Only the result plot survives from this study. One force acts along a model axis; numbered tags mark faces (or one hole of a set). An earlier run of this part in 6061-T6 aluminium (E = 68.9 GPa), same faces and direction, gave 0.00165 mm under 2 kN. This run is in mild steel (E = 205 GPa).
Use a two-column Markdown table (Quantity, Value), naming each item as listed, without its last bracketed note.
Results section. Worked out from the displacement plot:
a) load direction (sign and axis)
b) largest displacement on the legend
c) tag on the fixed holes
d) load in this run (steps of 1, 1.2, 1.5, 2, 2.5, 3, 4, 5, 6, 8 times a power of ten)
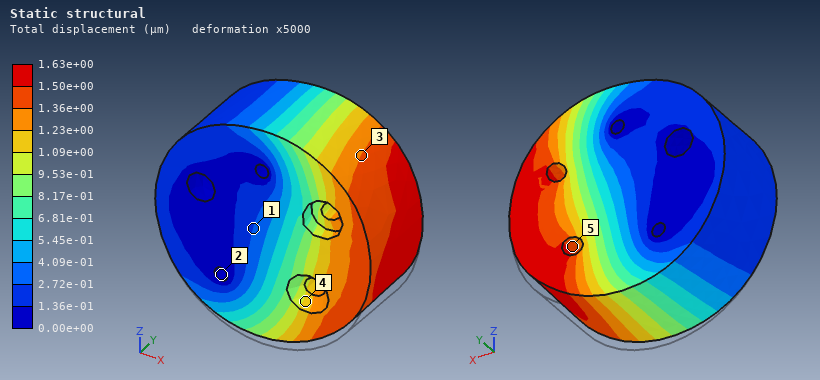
| Quantity | Value |
|---|---|
| load direction | +Z |
| largest displacement on the legend | 1.63e+00 µm |
| tag on the fixed holes | 2 |
| load in this run | 6 kN |
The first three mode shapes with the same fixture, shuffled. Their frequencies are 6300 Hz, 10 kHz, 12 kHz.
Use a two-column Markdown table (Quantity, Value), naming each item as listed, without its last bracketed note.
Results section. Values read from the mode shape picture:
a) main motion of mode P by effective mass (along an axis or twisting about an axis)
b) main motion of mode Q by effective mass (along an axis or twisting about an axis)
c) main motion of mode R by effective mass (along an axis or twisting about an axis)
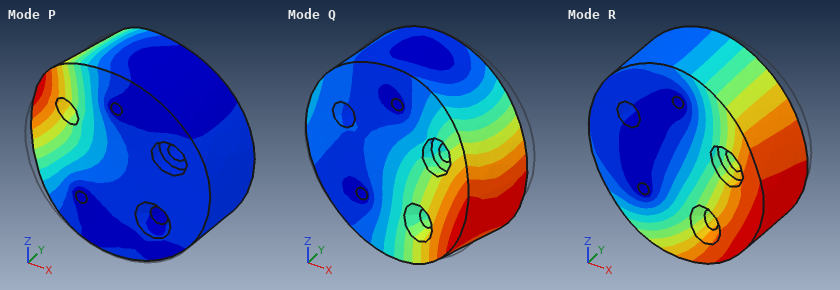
| Quantity | Value |
|---|---|
| main motion of mode P by effective mass | along Y |
| main motion of mode Q by effective mass | along Y |
| main motion of mode R by effective mass | along Z |
